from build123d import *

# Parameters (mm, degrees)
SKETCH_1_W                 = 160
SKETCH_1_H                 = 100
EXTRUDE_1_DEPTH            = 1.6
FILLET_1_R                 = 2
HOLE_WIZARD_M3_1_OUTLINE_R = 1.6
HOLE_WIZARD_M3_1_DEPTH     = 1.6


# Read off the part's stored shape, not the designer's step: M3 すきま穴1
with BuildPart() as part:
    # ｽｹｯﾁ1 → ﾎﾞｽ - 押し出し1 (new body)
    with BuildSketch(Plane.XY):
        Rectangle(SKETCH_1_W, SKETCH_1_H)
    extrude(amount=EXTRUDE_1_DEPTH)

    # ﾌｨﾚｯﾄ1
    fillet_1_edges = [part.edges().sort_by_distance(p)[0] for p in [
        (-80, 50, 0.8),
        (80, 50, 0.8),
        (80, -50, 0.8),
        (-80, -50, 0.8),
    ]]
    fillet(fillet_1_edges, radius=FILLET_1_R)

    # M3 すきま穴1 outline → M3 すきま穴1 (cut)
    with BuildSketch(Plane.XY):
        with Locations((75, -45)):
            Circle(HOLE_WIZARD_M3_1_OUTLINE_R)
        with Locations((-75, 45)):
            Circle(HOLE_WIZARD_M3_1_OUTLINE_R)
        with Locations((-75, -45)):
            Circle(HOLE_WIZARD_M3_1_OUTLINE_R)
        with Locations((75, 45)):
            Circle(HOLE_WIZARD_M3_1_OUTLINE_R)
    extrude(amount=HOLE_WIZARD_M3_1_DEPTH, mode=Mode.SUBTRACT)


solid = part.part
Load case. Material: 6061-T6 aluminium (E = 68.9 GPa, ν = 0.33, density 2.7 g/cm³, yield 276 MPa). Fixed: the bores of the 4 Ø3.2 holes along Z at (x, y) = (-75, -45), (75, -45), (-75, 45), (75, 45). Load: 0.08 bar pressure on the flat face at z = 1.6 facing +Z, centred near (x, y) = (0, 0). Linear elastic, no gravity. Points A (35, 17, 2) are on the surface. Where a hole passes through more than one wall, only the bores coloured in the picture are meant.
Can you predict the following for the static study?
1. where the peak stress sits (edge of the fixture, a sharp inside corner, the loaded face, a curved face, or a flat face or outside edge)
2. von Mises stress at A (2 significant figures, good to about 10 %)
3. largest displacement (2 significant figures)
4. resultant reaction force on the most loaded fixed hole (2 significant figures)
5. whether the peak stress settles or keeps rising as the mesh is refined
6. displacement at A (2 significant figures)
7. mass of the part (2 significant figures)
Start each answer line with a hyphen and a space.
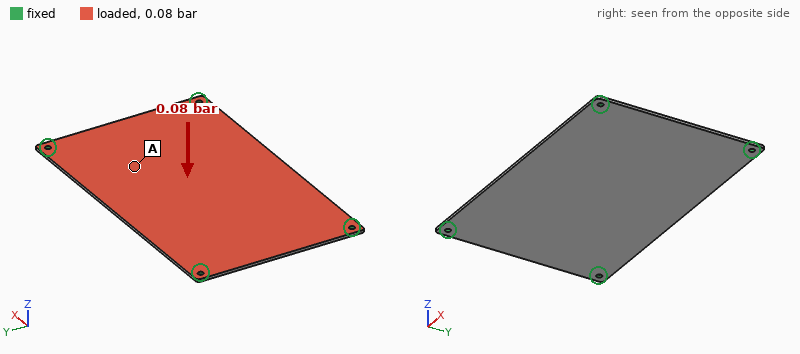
- edge of the fixture
- 12 MPa
- 0.74 mm
- 32 N
- keeps rising
- 0.52 mm
- 69 g
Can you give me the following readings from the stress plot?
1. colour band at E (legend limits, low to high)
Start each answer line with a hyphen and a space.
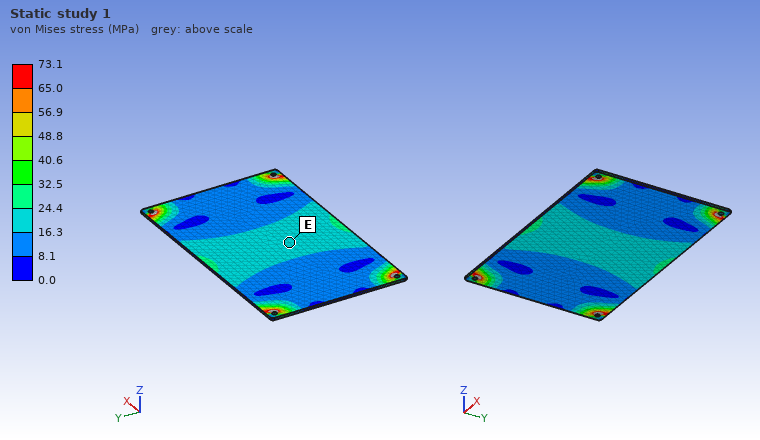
- 16.3 to 24.4 MPa
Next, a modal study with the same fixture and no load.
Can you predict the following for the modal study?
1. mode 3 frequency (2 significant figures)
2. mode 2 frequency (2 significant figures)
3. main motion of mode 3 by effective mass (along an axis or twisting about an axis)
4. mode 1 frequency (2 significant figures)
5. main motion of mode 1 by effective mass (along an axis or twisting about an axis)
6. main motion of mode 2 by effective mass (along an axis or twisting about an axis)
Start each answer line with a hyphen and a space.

- 760 Hz
- 510 Hz
- twisting about Y
- 290 Hz
- along Z
- twisting about X
